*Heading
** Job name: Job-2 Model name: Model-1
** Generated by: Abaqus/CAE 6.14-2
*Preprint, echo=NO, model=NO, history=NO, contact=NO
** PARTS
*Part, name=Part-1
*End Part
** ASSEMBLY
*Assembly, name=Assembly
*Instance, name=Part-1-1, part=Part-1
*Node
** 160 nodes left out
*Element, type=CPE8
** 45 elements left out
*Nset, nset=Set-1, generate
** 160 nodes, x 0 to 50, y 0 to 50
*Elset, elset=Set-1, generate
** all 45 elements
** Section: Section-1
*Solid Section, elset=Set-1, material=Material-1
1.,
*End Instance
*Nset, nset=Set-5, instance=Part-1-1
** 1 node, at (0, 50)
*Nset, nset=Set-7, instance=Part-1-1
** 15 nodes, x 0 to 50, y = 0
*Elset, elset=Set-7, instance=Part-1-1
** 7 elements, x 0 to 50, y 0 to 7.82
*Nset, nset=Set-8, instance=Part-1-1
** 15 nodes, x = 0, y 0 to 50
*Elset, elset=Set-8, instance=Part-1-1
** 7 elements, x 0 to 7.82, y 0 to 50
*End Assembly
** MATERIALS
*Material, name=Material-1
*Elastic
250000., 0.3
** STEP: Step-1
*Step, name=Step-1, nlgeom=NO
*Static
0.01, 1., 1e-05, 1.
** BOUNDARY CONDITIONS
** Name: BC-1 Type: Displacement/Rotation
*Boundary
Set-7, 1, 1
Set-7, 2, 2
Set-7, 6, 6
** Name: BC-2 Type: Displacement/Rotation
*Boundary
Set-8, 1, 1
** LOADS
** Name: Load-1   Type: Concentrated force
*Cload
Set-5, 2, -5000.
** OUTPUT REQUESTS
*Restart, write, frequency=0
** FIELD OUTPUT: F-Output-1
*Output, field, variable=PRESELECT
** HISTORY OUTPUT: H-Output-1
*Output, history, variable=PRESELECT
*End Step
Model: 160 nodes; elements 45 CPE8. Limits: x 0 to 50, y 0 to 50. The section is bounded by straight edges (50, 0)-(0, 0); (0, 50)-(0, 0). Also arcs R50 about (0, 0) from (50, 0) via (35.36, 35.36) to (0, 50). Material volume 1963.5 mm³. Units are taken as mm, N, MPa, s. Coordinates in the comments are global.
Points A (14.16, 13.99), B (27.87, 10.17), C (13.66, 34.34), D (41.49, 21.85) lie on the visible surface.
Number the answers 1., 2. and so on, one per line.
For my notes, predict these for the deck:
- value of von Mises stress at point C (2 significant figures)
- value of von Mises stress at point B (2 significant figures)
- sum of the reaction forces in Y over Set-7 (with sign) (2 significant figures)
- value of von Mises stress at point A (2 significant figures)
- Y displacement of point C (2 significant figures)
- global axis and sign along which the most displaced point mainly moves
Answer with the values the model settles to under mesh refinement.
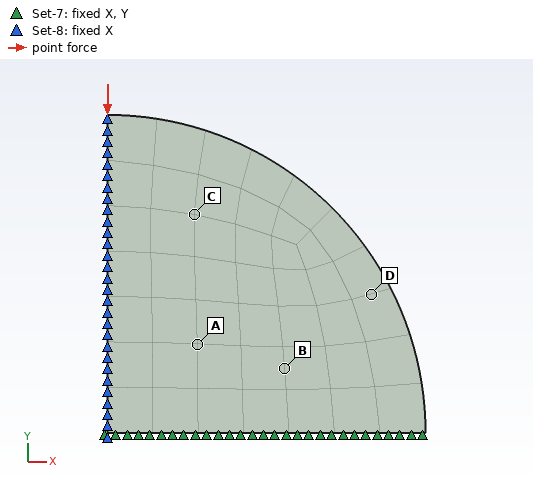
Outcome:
1. 200 MPa
2. 88 MPa
3. 5000 N
4. 150 MPa
5. -0.018 mm
6. -Y
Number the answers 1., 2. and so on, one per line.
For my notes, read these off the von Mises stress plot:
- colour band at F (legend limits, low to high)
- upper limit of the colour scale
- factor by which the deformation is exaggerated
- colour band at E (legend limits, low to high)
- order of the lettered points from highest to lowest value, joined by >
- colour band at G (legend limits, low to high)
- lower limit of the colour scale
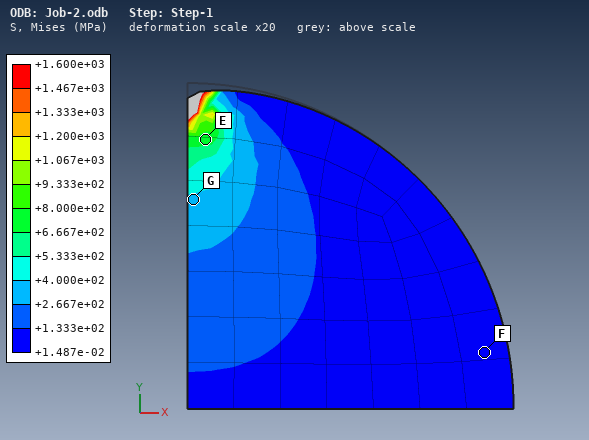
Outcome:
1. +1.487e-02 to +1.333e+02 MPa
2. +1.600e+03 MPa
3. 20
4. +6.667e+02 to +8.000e+02 MPa
5. E > G > F
6. +2.667e+02 to +4.000e+02 MPa
7. +1.487e-02 MPa
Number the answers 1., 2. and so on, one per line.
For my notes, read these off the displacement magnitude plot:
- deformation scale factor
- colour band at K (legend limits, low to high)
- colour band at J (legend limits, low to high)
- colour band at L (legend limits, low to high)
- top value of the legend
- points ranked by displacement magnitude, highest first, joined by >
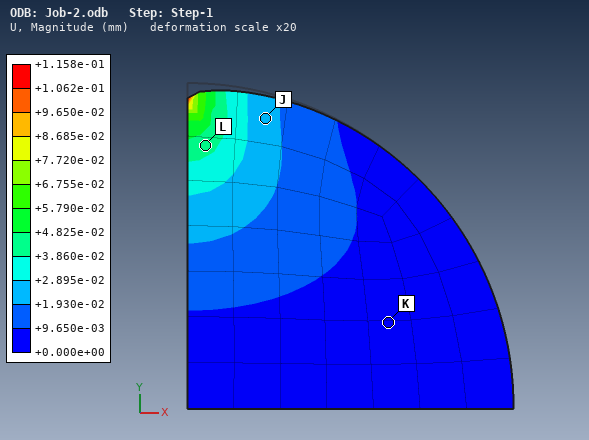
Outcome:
1. 20
2. +0.000e+00 to +9.650e-03 mm
3. +1.930e-02 to +2.895e-02 mm
4. +3.860e-02 to +4.825e-02 mm
5. +1.158e-01 mm
6. L > J > K
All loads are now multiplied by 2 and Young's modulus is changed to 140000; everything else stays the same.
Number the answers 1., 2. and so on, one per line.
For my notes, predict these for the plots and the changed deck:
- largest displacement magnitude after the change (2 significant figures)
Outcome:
1. 0.41 mm
